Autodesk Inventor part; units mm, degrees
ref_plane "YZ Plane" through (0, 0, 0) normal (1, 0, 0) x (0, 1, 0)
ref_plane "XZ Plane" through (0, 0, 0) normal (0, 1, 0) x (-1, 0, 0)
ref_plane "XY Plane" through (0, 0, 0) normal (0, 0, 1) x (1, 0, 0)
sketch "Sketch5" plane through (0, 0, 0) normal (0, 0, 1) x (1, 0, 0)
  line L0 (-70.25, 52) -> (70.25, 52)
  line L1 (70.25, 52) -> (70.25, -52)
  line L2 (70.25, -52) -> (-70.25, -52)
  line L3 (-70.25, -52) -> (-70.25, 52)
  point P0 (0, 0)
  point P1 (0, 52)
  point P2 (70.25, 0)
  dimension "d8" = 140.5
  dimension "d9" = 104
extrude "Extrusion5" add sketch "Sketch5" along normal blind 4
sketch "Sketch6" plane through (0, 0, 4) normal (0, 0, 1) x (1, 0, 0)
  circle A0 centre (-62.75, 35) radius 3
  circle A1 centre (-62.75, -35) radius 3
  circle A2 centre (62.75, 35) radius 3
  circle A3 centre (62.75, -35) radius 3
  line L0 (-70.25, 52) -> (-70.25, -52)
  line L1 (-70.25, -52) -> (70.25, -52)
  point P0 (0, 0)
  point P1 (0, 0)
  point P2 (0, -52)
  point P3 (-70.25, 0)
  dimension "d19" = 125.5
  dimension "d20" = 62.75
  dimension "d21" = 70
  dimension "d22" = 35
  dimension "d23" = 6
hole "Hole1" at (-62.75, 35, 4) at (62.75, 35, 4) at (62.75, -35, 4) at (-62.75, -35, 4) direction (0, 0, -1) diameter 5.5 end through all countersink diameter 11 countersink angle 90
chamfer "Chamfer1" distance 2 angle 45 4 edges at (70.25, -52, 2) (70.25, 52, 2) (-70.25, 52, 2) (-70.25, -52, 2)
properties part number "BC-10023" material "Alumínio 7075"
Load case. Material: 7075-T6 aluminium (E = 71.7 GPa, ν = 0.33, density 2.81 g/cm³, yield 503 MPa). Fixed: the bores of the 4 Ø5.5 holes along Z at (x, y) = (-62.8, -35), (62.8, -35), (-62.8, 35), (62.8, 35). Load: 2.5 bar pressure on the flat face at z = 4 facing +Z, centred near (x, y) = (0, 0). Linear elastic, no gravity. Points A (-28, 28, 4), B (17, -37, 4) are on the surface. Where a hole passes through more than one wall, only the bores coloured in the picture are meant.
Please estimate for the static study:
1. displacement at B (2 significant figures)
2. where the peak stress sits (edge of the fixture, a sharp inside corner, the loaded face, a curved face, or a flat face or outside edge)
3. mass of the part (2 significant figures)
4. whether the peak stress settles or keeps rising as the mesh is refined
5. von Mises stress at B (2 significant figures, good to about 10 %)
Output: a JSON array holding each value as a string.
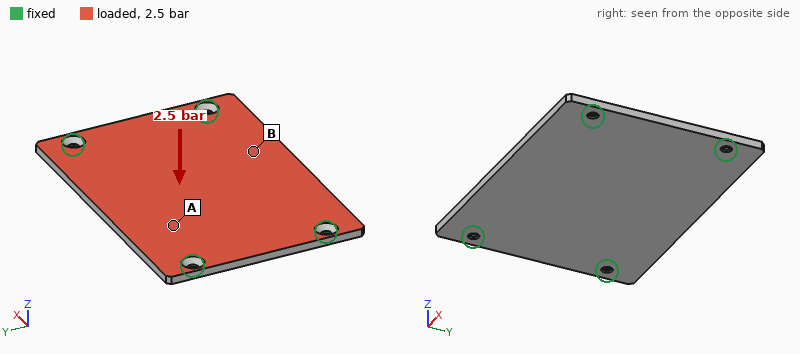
["0.66 mm", "edge of the fixture", "160 g", "keeps rising", "82 MPa"]
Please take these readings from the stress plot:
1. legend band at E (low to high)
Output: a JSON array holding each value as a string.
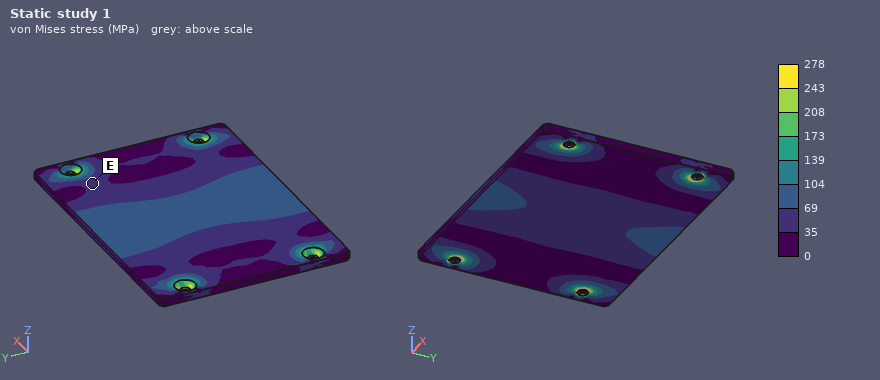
["35 to 69 MPa"]
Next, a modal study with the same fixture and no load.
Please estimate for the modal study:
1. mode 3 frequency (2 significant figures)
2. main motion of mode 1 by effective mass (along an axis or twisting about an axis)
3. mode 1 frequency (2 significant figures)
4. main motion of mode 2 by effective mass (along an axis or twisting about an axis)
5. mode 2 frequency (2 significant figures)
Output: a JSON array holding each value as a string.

["2500 Hz", "along Z", "980 Hz", "twisting about X", "1400 Hz"]
